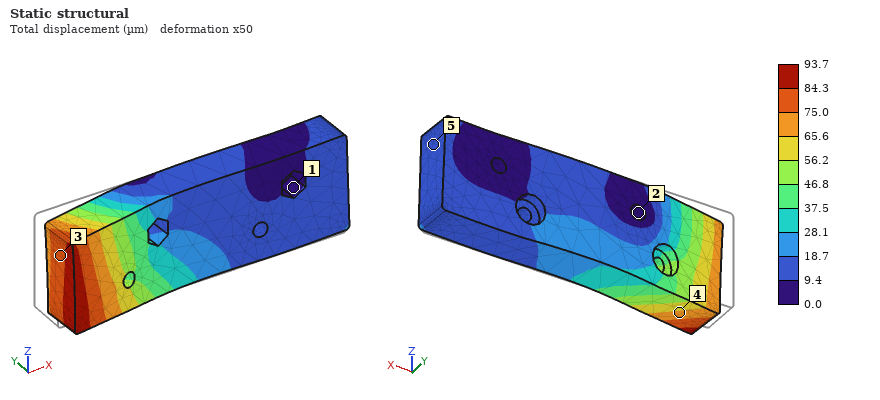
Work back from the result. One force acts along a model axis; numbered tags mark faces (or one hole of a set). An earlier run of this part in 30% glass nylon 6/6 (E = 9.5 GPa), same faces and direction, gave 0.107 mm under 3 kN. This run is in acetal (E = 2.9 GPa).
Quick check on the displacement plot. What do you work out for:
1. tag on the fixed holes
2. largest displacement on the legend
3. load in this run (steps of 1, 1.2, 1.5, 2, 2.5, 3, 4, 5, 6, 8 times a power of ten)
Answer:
2
93.7 µm
800 N
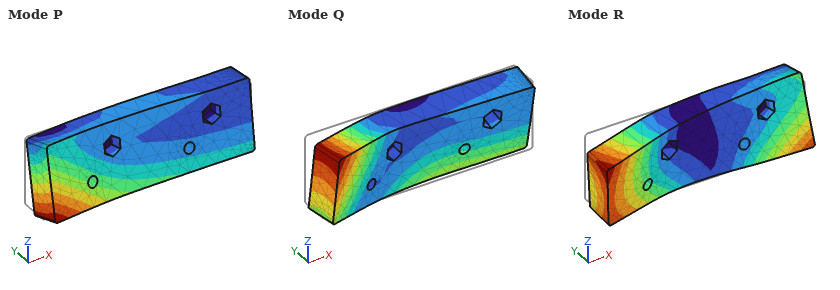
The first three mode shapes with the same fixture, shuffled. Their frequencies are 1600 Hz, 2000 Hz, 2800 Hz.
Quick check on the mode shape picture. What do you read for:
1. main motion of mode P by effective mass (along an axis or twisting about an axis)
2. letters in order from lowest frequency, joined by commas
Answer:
along Y
P, Q, R
